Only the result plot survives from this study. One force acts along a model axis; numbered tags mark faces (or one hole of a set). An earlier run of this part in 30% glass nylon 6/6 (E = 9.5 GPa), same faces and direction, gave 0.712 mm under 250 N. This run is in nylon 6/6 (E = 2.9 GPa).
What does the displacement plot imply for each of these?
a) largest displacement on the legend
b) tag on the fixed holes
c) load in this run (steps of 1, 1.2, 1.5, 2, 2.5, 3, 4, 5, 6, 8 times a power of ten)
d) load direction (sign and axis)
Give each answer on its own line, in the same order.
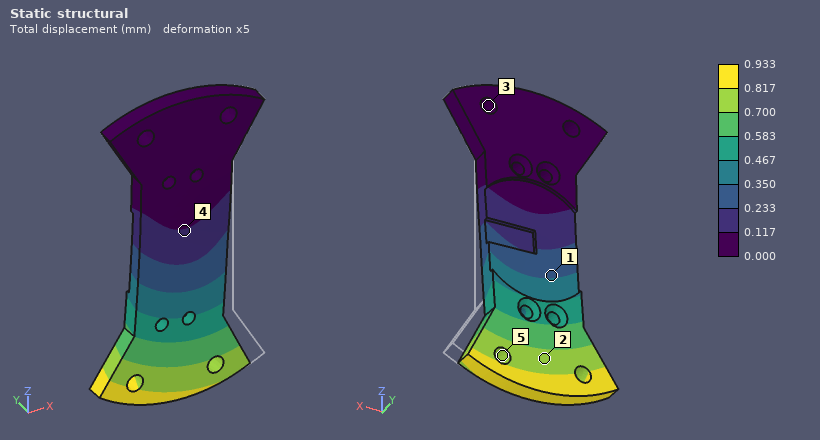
0.933 mm
3
100 N
-X
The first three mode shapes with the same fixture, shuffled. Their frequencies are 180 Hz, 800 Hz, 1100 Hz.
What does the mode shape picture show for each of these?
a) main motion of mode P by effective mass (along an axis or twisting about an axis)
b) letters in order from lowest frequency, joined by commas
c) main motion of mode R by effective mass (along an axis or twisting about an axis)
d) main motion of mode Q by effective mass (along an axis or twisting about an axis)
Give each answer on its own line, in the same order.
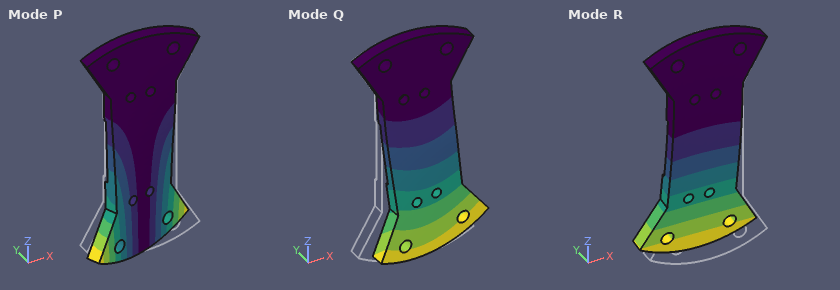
twisting about Z
R, P, Q
along Y
along X
